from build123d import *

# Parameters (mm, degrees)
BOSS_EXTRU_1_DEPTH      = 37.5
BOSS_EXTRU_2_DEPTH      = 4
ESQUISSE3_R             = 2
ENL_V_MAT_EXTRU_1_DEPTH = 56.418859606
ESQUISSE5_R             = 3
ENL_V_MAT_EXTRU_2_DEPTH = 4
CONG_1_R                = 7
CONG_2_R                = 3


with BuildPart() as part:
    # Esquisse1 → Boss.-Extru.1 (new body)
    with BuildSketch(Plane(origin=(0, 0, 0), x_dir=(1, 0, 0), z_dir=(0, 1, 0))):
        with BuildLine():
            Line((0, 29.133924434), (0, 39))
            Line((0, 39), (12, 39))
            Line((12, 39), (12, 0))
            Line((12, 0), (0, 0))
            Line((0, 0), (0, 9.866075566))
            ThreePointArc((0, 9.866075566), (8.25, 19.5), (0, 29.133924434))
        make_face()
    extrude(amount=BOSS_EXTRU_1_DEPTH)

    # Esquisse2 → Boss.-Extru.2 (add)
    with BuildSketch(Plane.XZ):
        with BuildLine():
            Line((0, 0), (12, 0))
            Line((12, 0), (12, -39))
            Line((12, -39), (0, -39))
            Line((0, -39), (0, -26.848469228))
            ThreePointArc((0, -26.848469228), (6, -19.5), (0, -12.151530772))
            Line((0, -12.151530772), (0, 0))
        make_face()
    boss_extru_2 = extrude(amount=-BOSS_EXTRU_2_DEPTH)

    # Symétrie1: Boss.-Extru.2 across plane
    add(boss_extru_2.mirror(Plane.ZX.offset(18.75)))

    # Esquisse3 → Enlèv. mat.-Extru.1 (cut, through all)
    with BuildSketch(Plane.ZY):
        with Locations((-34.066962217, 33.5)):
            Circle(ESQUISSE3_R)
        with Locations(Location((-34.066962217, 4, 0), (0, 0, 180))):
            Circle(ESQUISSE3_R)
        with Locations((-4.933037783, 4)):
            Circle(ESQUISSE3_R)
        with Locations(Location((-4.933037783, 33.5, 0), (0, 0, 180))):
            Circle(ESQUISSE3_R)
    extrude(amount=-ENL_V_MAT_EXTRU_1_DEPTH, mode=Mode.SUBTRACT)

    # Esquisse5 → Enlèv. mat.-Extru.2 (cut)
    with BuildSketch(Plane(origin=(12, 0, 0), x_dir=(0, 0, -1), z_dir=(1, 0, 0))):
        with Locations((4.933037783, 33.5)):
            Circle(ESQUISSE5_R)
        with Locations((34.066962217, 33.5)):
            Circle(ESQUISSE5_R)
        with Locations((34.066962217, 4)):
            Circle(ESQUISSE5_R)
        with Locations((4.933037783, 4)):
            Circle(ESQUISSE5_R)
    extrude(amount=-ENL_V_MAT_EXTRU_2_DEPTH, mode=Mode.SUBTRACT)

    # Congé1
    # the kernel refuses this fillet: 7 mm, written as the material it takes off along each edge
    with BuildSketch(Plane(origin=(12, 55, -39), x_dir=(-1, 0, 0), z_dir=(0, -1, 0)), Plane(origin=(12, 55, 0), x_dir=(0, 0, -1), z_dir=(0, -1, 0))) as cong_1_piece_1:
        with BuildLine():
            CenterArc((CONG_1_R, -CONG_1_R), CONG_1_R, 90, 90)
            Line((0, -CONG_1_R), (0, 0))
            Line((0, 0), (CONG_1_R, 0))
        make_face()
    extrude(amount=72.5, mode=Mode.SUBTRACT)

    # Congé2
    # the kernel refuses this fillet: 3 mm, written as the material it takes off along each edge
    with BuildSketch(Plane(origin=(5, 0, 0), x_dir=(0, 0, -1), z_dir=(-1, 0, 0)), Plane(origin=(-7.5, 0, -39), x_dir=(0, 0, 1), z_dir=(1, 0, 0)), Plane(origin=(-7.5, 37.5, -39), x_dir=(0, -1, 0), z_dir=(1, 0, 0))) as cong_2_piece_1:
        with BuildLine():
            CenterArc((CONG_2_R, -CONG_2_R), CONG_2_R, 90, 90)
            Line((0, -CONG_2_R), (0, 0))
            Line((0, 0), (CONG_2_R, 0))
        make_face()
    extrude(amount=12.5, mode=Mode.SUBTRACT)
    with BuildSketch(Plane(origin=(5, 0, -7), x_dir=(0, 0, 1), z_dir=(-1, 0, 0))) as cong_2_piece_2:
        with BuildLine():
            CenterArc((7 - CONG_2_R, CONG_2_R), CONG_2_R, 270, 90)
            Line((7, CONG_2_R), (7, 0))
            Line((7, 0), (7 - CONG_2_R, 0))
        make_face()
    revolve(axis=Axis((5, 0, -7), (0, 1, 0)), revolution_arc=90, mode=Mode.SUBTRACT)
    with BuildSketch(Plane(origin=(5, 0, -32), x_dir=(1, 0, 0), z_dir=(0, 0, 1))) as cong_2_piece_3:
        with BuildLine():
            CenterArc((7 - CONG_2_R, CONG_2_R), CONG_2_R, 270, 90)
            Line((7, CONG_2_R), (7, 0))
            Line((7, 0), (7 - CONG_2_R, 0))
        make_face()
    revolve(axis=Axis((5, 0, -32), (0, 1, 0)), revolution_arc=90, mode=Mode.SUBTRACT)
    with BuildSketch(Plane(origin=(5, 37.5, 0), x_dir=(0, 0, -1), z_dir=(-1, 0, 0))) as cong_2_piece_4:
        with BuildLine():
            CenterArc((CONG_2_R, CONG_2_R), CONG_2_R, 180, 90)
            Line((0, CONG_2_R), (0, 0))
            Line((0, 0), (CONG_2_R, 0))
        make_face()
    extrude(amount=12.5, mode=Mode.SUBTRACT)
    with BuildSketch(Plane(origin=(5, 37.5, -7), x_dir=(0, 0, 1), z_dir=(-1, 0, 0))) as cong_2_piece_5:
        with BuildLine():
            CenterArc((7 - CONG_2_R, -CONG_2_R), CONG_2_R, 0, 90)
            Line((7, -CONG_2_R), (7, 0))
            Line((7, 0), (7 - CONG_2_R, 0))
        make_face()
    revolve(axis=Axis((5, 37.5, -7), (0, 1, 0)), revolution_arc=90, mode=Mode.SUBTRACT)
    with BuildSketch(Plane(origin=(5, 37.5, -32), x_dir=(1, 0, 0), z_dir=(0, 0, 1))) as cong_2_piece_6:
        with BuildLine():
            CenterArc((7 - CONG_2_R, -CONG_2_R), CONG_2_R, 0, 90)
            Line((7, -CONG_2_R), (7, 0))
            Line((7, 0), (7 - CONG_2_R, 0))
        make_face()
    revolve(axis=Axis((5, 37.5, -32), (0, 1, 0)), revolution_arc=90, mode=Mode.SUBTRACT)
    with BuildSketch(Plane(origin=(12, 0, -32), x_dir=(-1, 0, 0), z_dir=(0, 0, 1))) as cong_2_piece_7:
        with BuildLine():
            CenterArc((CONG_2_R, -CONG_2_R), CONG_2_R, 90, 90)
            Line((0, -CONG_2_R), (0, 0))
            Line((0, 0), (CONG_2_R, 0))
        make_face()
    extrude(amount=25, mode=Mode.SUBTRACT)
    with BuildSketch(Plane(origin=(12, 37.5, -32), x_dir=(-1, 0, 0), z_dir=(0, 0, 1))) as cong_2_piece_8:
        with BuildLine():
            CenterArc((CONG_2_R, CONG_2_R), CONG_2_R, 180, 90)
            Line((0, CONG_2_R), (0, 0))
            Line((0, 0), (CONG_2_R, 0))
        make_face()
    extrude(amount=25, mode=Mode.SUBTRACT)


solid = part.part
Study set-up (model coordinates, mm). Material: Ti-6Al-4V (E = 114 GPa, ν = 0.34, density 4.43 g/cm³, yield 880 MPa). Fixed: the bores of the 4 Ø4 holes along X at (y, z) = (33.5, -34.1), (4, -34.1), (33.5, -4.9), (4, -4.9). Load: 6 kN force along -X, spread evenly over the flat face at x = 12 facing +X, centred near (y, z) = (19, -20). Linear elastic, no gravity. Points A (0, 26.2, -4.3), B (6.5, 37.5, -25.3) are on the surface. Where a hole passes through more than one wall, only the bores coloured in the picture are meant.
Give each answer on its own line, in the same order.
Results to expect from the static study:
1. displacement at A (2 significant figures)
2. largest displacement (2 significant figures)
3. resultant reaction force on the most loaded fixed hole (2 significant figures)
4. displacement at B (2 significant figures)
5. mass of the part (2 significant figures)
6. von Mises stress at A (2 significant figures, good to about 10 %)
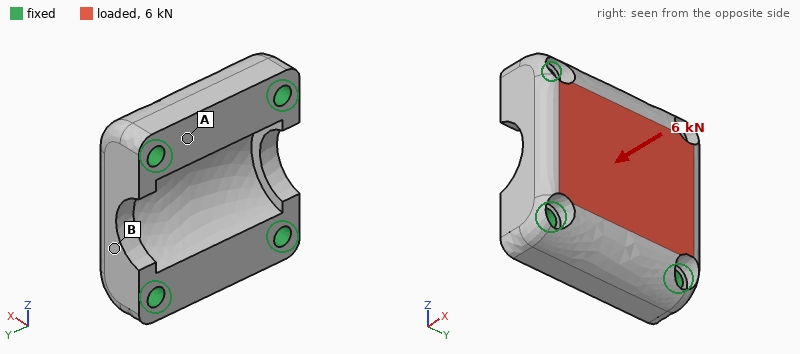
3.0 µm
9.4 µm
2.0 kN
2.1 µm
52 g
16 MPa
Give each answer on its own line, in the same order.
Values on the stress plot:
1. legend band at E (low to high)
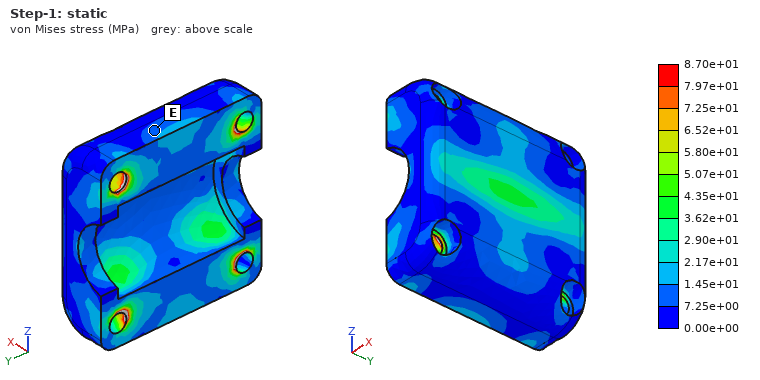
7.25e+00 to 1.45e+01 MPa
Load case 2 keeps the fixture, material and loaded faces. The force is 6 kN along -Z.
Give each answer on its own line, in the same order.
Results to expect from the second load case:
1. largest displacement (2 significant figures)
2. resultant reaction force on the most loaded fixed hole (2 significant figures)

4.2 µm
1.7 kN
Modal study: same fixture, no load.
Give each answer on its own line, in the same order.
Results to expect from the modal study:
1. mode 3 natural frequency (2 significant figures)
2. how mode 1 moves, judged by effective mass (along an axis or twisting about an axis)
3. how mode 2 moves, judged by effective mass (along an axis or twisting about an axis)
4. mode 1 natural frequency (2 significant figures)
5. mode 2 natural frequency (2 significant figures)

40 kHz
along X
along Z
31 kHz
35 kHz
